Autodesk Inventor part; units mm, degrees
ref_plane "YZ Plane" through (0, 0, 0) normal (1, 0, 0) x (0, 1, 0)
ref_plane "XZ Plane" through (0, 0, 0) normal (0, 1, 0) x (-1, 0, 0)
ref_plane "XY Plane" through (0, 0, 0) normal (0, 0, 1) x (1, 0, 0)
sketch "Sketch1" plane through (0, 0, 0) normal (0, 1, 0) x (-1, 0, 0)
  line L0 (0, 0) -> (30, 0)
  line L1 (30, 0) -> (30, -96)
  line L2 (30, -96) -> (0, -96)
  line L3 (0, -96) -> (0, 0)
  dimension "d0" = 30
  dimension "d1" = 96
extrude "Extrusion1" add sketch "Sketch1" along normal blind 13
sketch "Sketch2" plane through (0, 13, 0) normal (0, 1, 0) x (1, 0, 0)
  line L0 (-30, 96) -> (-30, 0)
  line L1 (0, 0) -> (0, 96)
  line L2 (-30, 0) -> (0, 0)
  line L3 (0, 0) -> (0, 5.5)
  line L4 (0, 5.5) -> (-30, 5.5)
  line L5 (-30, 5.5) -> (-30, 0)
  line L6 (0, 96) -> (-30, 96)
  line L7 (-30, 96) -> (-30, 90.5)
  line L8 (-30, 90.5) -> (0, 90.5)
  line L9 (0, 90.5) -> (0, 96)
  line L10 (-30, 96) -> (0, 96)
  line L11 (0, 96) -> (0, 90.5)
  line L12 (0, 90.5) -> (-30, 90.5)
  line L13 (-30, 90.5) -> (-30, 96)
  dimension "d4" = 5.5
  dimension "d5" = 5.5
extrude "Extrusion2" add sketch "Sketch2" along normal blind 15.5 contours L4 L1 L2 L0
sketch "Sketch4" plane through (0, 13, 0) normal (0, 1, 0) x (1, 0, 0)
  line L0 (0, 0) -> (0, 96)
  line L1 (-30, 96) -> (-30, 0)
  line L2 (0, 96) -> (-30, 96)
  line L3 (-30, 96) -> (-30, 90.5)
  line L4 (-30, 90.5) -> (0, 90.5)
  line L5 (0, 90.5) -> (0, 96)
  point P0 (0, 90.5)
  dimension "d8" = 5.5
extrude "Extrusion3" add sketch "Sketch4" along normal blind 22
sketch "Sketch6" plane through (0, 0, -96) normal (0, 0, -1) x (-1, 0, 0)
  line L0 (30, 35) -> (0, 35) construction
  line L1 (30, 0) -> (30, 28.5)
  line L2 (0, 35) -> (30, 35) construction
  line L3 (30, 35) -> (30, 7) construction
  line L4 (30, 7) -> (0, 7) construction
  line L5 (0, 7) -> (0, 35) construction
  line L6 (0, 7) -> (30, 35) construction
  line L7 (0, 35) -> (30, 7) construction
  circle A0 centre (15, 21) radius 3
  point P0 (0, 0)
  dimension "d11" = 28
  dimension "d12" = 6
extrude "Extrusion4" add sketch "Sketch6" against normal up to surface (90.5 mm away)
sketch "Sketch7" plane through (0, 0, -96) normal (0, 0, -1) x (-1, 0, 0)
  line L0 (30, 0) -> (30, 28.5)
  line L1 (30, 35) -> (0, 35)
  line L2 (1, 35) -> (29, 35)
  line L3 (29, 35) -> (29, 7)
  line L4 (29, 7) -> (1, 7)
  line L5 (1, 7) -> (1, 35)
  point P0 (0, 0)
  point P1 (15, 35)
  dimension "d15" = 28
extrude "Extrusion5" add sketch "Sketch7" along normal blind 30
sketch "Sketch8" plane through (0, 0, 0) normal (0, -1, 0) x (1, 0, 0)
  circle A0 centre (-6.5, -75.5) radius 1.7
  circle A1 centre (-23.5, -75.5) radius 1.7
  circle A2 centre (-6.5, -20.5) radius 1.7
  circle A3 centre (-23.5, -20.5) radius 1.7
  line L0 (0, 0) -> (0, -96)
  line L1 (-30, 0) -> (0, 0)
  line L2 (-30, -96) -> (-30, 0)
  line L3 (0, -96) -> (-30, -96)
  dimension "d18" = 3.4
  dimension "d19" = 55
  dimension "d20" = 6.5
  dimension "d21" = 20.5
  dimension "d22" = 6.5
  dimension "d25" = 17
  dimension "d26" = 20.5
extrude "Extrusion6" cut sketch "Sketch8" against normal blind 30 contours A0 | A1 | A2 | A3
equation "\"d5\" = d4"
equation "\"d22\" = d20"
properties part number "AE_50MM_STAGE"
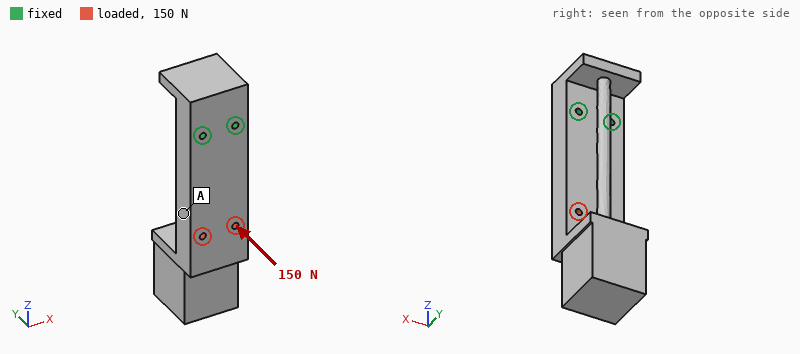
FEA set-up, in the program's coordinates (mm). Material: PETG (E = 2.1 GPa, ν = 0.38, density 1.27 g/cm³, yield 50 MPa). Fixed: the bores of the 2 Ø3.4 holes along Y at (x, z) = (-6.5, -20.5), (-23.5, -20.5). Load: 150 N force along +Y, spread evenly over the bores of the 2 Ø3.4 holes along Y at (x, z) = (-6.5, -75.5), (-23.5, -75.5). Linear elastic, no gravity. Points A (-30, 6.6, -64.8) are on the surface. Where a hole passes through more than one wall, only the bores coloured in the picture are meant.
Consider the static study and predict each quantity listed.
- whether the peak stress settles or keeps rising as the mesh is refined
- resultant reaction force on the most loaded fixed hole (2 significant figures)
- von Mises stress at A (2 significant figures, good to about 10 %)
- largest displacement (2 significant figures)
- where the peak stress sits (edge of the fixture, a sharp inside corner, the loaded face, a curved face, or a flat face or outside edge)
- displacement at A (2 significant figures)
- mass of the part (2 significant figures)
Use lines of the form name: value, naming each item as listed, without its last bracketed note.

whether the peak stress settles or keeps rising as the mesh is refined: keeps rising
resultant reaction force on the most loaded fixed hole: 77 N
von Mises stress at A: 1.6 MPa
largest displacement: 1.4 mm
where the peak stress sits: edge of the fixture
displacement at A: 0.49 mm
mass of the part: 88 g
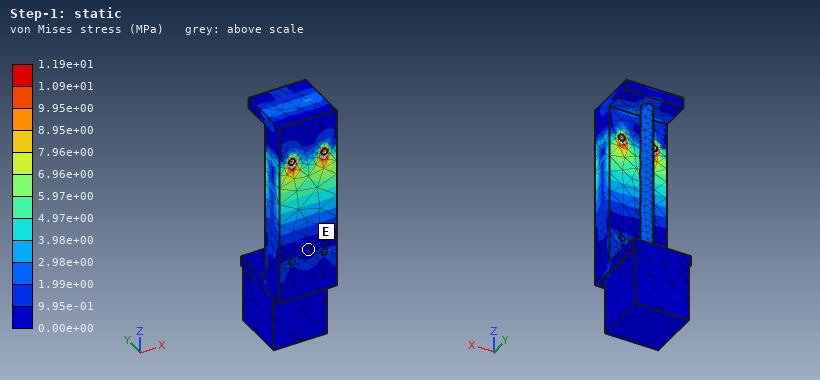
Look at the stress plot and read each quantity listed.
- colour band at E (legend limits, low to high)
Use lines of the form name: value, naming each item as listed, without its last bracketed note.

colour band at E: 0.00e+00 to 9.95e-01 MPa
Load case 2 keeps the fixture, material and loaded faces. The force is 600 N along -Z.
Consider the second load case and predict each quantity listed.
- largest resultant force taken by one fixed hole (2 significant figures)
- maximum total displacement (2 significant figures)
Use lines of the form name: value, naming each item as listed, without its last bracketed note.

largest resultant force taken by one fixed hole: 300 N
maximum total displacement: 80 µm
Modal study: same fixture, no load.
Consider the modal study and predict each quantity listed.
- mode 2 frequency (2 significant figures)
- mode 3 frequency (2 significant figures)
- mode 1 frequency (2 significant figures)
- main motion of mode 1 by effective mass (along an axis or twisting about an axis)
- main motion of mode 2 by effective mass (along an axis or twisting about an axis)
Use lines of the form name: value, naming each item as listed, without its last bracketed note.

mode 2 frequency: 330 Hz
mode 3 frequency: 820 Hz
mode 1 frequency: 200 Hz
main motion of mode 1 by effective mass: along Y
main motion of mode 2 by effective mass: along X
